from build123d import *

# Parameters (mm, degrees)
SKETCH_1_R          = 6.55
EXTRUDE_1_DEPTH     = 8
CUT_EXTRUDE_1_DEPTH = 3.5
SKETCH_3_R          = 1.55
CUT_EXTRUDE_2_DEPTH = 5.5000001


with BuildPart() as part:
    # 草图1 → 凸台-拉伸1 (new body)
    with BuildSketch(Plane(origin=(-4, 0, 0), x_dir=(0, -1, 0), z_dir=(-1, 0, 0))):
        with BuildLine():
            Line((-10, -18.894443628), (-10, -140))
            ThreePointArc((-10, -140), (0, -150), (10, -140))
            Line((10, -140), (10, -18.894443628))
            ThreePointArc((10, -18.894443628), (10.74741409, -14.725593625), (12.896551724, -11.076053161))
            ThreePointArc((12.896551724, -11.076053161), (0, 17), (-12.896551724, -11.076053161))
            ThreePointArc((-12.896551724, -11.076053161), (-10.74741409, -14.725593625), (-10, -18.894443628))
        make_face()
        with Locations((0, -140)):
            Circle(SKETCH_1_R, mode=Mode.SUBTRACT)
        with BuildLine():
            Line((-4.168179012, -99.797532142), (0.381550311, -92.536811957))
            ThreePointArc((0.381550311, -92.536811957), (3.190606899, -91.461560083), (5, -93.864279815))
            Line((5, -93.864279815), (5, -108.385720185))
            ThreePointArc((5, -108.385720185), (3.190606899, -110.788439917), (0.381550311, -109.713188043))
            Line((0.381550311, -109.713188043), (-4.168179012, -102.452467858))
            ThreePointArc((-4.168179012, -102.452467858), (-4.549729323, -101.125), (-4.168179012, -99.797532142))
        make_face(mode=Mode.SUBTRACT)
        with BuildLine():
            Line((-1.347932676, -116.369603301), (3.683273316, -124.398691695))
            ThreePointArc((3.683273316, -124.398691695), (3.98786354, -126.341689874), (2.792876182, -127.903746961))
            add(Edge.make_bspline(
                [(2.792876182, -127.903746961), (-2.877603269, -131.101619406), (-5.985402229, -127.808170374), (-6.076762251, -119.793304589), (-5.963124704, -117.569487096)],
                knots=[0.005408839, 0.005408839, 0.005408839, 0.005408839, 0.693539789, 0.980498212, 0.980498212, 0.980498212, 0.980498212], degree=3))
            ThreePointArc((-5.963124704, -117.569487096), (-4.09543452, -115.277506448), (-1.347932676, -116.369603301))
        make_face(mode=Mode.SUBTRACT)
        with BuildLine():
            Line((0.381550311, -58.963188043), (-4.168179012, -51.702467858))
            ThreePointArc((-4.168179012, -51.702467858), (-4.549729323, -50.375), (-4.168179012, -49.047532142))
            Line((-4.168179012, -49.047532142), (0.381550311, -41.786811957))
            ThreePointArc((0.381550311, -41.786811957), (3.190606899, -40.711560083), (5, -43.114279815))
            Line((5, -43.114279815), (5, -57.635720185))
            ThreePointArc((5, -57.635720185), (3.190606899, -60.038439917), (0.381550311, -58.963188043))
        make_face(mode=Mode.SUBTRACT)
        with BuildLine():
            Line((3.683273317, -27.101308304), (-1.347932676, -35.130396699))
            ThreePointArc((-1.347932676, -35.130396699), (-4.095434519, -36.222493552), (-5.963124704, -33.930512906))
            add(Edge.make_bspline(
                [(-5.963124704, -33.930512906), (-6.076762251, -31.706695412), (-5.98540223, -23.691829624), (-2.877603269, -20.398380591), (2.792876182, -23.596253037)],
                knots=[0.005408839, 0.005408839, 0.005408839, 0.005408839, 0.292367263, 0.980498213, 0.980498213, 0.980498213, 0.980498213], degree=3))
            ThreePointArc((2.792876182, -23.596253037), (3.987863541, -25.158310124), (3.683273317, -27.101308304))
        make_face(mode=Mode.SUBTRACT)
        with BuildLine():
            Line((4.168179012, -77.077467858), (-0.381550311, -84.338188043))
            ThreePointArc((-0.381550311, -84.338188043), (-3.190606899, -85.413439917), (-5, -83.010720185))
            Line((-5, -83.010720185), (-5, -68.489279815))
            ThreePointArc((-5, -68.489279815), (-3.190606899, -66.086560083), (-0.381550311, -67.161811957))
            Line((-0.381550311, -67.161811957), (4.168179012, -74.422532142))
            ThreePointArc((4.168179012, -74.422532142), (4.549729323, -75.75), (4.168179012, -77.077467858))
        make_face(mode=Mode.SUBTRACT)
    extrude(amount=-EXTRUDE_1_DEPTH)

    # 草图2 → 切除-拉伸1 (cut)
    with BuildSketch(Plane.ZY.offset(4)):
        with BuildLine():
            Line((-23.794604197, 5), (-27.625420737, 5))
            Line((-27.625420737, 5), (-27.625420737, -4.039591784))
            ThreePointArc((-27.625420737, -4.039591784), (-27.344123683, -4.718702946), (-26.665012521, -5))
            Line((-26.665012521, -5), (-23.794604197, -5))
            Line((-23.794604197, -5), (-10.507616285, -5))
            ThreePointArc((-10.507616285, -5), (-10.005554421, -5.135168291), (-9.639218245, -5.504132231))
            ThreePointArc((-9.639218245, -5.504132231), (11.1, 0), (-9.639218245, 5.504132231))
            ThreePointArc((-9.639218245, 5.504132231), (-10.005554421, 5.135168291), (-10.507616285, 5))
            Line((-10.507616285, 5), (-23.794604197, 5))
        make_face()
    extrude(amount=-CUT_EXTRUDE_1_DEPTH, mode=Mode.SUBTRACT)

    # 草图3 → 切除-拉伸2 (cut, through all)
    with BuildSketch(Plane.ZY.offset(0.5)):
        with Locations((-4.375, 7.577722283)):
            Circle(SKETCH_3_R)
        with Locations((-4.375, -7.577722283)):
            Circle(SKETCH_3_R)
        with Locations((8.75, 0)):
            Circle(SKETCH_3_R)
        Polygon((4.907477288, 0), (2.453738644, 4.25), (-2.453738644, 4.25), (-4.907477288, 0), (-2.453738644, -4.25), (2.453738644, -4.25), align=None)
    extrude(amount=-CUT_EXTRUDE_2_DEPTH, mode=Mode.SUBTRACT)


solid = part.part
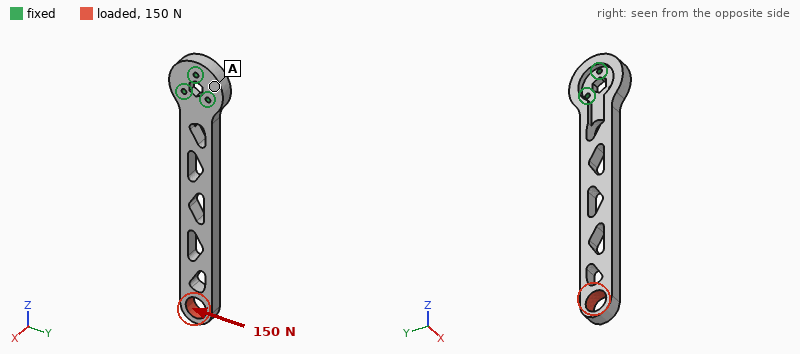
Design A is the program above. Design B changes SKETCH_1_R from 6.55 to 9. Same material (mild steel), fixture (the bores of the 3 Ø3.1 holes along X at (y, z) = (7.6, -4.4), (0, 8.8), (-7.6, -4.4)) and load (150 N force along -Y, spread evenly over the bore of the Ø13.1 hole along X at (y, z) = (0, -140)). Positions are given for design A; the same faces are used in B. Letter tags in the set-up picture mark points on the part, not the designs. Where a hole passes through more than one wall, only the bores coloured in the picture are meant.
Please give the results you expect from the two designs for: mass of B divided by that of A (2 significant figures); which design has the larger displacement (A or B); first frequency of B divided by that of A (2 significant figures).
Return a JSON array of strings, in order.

["0.95", "B", "1.1"]
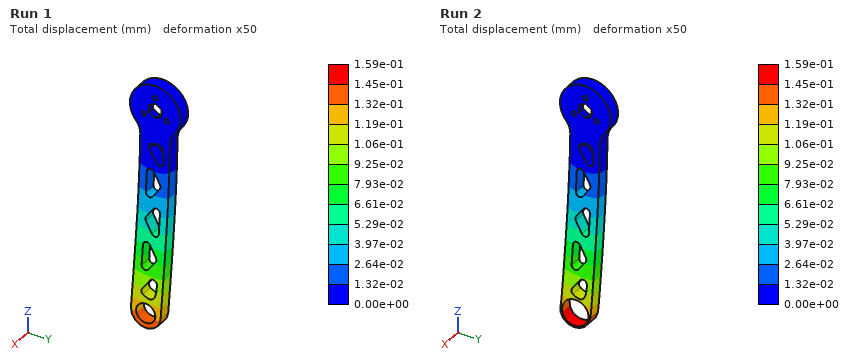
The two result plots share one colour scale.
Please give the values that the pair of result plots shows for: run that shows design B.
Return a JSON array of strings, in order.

["Run 2"]
